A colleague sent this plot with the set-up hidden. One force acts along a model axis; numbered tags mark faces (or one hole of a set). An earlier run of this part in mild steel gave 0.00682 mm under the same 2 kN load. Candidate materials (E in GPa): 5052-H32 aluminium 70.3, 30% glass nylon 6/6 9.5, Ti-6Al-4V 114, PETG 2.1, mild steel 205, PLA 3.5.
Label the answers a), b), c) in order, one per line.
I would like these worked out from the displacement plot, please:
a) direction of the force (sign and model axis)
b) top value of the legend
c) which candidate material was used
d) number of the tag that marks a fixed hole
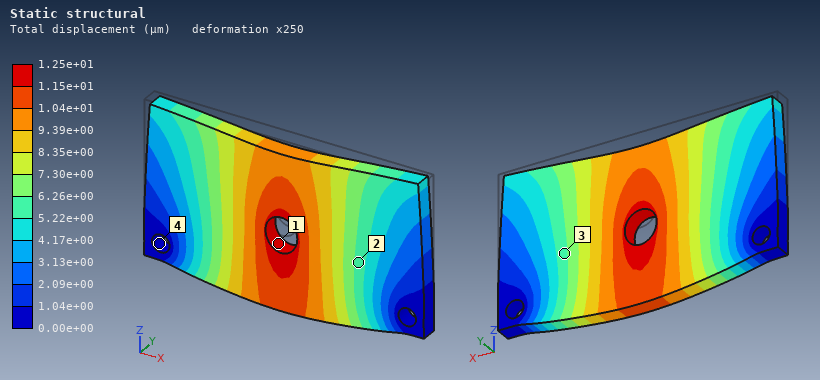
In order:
a) -Z
b) 1.25e+01 µm
c) Ti-6Al-4V
d) 4
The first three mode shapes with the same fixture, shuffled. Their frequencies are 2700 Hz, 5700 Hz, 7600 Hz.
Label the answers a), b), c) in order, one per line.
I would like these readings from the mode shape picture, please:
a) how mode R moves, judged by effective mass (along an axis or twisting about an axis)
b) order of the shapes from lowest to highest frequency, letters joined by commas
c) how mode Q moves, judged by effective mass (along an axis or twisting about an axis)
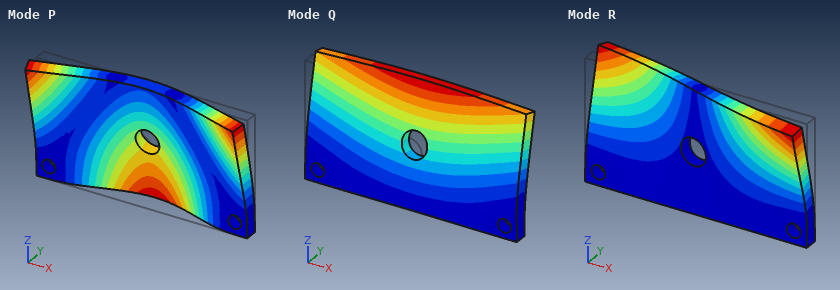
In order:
a) twisting about Z
b) Q, R, P
c) along Y
